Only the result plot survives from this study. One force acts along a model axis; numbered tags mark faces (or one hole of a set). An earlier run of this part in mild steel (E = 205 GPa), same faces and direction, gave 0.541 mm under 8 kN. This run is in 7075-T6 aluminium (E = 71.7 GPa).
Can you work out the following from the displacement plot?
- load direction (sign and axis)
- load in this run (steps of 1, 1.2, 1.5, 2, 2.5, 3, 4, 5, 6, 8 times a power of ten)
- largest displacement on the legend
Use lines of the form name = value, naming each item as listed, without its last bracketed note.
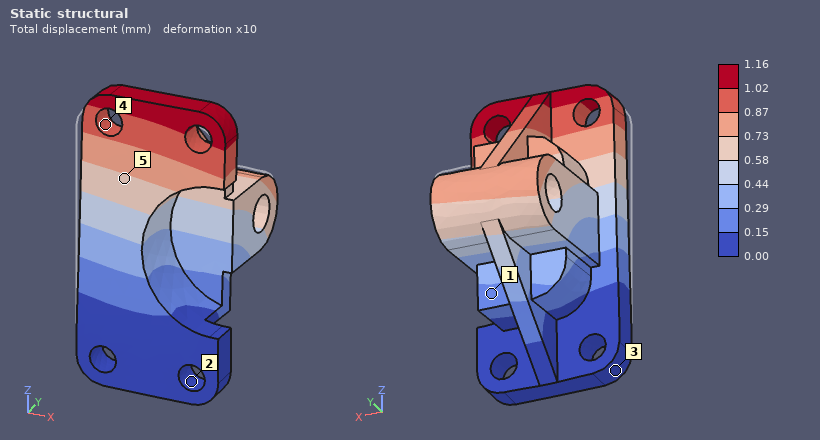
load direction = +Y
load in this run = 6 kN
largest displacement on the legend = 1.16 mm
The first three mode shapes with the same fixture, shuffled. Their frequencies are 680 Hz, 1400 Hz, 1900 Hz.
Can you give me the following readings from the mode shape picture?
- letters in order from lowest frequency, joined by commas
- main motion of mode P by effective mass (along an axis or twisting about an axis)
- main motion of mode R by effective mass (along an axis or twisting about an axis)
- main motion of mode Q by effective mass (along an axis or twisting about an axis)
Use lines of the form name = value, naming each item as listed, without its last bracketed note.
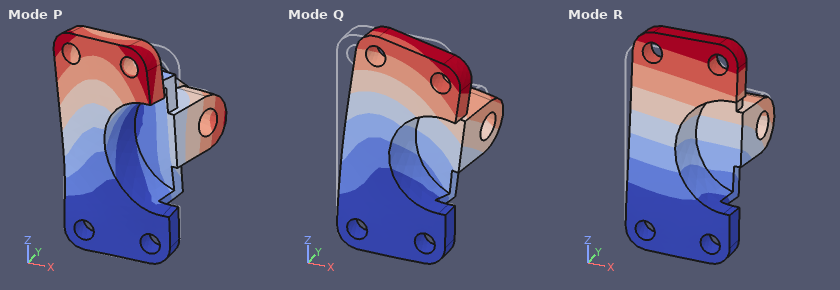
letters in order from lowest frequency, joined by commas = R, Q, P
main motion of mode P by effective mass = twisting about Z
main motion of mode R by effective mass = along Y
main motion of mode Q by effective mass = along X
